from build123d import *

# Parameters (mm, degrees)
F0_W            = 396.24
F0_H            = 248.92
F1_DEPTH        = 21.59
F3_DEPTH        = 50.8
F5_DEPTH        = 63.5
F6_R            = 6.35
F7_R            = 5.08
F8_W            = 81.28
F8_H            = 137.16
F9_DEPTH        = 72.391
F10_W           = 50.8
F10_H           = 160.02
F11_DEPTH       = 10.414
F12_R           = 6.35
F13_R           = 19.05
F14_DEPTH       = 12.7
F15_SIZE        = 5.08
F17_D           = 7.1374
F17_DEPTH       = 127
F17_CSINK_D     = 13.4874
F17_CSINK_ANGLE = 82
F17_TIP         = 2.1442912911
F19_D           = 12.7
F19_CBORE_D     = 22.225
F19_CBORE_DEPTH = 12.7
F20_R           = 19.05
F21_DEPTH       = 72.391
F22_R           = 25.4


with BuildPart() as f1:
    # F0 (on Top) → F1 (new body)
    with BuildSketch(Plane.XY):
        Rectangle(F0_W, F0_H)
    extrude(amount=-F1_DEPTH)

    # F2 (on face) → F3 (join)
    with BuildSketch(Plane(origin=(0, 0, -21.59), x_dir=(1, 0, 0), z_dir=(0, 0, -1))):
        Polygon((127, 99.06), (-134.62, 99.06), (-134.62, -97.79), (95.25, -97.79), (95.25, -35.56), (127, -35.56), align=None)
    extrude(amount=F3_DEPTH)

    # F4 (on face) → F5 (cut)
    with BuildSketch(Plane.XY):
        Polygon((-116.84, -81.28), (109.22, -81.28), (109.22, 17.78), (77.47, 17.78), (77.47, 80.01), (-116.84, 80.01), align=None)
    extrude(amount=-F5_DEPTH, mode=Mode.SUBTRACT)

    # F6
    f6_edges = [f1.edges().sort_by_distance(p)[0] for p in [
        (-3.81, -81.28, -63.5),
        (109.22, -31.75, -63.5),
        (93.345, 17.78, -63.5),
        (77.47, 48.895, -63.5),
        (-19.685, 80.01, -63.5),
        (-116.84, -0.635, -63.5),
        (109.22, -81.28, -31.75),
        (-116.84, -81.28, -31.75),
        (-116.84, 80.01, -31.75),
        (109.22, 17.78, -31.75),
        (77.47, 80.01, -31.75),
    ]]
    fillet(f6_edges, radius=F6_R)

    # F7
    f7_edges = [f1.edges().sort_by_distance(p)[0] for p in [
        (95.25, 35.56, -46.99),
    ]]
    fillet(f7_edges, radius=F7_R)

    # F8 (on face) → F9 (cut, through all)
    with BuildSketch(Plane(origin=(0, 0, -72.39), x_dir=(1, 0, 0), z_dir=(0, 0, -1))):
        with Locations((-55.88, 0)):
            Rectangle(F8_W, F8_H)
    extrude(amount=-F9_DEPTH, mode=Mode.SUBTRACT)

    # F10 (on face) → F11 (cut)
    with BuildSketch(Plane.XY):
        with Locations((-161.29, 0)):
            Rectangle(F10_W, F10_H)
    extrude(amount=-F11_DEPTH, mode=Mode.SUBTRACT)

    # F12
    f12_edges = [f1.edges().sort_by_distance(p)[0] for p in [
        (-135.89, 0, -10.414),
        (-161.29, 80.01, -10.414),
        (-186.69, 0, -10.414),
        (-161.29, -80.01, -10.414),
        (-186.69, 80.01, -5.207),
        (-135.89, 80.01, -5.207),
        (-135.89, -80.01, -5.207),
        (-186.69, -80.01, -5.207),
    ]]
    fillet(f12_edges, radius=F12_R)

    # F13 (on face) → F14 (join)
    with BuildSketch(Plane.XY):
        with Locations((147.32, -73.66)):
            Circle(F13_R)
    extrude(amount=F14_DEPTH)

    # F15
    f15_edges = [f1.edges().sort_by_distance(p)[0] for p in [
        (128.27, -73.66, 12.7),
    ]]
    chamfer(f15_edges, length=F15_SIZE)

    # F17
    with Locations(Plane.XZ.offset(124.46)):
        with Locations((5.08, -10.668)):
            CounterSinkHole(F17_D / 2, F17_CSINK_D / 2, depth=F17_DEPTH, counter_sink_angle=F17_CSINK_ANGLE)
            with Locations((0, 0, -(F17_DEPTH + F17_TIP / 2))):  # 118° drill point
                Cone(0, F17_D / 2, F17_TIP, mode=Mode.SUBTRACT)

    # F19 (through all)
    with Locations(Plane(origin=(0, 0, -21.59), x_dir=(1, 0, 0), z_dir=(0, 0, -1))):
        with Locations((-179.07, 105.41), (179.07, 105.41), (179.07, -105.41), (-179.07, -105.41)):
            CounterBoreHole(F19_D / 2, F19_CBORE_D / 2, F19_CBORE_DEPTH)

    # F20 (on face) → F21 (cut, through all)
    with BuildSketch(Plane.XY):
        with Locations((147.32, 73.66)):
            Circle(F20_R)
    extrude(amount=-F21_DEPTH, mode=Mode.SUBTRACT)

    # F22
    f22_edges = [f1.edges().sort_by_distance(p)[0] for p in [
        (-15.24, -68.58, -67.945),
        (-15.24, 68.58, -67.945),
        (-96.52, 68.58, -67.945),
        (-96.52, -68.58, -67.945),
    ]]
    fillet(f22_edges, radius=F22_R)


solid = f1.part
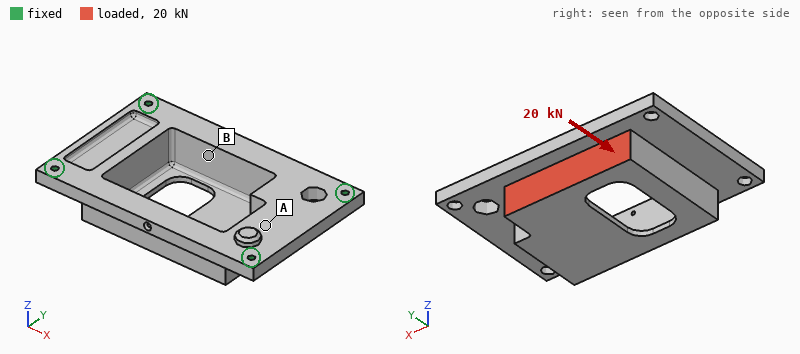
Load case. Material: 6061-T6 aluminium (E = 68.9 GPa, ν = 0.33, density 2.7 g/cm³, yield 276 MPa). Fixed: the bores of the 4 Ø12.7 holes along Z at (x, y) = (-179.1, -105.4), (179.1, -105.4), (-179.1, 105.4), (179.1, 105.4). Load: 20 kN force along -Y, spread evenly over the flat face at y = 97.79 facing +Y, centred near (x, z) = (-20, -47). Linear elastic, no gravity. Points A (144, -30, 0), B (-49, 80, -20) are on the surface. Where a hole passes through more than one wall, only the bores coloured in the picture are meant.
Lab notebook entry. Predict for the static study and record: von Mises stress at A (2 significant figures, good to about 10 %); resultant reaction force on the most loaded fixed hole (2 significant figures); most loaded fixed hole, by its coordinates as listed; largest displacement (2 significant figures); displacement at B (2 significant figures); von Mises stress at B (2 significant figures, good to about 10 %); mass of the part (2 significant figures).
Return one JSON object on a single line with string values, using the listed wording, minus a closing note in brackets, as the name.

{"von Mises stress at A": "3.5 MPa", "resultant reaction force on the most loaded fixed hole": "8.2 kN", "most loaded fixed hole, by its coordinates as listed": "(179.1, -105.4)", "largest displacement": "72 µm", "displacement at B": "54 µm", "von Mises stress at B": "8.1 MPa", "mass of the part": "6.1 kg"}
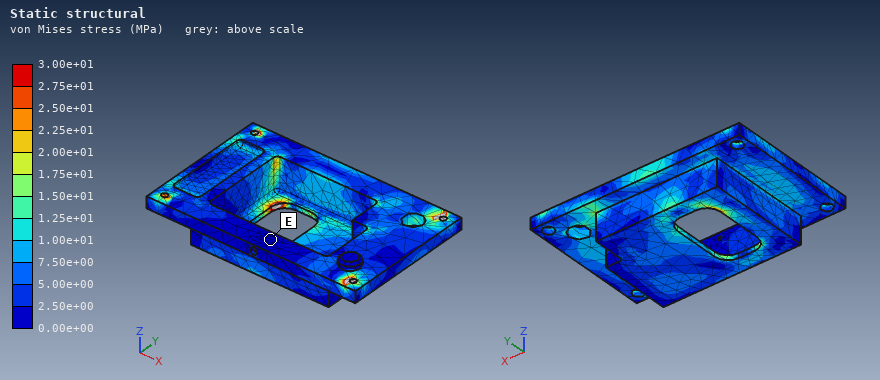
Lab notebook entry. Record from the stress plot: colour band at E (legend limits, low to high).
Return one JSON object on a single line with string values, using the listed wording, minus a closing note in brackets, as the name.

{"colour band at E": "0.00e+00 to 2.50e+00 MPa"}
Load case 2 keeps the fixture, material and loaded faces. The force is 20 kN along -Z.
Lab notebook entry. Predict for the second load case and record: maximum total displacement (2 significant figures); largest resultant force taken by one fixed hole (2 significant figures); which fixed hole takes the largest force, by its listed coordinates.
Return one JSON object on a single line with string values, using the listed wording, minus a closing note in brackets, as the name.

{"maximum total displacement": "0.33 mm", "largest resultant force taken by one fixed hole": "19 kN", "which fixed hole takes the largest force, by its listed coordinates": "(-179.1, 105.4)"}
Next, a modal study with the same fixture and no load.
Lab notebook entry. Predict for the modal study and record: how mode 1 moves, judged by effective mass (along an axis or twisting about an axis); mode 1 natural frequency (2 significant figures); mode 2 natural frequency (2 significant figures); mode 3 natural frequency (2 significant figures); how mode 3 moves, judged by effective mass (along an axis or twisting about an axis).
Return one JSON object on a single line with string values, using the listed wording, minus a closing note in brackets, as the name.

{"how mode 1 moves, judged by effective mass": "along Z", "mode 1 natural frequency": "970 Hz", "mode 2 natural frequency": "1300 Hz", "mode 3 natural frequency": "1700 Hz", "how mode 3 moves, judged by effective mass": "twisting about Y"}
